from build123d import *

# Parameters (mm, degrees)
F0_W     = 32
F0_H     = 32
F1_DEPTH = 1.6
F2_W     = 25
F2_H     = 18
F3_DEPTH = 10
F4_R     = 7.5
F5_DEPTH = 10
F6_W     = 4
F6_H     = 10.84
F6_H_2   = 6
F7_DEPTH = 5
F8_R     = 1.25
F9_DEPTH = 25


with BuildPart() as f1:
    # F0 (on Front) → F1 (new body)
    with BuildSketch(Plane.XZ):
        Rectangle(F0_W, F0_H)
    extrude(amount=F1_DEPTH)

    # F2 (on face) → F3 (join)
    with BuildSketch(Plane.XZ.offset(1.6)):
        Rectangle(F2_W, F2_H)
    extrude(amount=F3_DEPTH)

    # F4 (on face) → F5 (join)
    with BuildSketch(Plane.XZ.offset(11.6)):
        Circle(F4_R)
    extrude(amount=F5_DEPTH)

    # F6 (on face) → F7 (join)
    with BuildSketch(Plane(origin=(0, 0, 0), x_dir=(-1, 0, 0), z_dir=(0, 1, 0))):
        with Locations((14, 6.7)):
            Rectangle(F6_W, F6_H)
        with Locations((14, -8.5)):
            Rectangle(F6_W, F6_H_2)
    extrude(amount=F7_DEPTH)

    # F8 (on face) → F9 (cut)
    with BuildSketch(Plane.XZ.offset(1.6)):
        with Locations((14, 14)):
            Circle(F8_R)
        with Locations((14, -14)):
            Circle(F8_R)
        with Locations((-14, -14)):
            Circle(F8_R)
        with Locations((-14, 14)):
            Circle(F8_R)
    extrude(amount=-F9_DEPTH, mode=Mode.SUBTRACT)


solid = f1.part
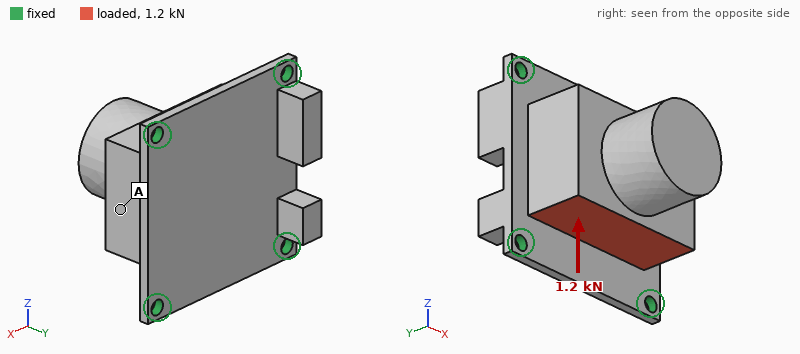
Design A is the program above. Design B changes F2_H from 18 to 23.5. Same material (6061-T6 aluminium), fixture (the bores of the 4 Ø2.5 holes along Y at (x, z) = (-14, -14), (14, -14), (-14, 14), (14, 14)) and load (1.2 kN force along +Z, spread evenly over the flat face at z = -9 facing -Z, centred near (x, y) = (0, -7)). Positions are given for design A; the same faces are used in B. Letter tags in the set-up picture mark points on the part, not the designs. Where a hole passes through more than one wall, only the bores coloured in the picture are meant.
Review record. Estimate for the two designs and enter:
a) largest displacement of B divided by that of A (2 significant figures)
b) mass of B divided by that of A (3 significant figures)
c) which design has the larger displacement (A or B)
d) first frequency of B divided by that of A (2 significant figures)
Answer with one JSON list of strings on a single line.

["0.39", "1.17", "A", "1.5"]
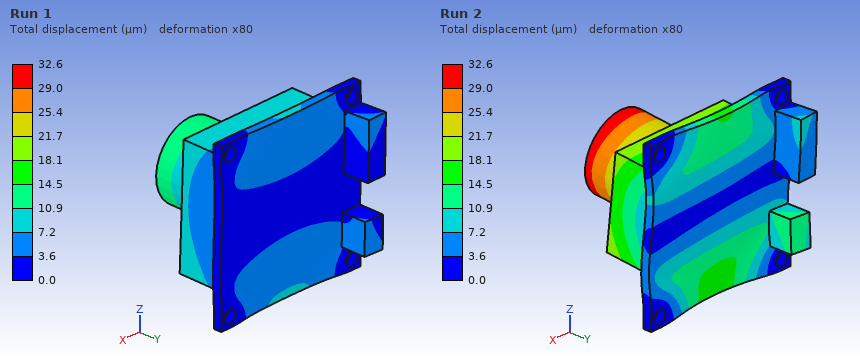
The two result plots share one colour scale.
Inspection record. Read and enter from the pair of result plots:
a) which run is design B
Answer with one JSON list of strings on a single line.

["Run 1"]
